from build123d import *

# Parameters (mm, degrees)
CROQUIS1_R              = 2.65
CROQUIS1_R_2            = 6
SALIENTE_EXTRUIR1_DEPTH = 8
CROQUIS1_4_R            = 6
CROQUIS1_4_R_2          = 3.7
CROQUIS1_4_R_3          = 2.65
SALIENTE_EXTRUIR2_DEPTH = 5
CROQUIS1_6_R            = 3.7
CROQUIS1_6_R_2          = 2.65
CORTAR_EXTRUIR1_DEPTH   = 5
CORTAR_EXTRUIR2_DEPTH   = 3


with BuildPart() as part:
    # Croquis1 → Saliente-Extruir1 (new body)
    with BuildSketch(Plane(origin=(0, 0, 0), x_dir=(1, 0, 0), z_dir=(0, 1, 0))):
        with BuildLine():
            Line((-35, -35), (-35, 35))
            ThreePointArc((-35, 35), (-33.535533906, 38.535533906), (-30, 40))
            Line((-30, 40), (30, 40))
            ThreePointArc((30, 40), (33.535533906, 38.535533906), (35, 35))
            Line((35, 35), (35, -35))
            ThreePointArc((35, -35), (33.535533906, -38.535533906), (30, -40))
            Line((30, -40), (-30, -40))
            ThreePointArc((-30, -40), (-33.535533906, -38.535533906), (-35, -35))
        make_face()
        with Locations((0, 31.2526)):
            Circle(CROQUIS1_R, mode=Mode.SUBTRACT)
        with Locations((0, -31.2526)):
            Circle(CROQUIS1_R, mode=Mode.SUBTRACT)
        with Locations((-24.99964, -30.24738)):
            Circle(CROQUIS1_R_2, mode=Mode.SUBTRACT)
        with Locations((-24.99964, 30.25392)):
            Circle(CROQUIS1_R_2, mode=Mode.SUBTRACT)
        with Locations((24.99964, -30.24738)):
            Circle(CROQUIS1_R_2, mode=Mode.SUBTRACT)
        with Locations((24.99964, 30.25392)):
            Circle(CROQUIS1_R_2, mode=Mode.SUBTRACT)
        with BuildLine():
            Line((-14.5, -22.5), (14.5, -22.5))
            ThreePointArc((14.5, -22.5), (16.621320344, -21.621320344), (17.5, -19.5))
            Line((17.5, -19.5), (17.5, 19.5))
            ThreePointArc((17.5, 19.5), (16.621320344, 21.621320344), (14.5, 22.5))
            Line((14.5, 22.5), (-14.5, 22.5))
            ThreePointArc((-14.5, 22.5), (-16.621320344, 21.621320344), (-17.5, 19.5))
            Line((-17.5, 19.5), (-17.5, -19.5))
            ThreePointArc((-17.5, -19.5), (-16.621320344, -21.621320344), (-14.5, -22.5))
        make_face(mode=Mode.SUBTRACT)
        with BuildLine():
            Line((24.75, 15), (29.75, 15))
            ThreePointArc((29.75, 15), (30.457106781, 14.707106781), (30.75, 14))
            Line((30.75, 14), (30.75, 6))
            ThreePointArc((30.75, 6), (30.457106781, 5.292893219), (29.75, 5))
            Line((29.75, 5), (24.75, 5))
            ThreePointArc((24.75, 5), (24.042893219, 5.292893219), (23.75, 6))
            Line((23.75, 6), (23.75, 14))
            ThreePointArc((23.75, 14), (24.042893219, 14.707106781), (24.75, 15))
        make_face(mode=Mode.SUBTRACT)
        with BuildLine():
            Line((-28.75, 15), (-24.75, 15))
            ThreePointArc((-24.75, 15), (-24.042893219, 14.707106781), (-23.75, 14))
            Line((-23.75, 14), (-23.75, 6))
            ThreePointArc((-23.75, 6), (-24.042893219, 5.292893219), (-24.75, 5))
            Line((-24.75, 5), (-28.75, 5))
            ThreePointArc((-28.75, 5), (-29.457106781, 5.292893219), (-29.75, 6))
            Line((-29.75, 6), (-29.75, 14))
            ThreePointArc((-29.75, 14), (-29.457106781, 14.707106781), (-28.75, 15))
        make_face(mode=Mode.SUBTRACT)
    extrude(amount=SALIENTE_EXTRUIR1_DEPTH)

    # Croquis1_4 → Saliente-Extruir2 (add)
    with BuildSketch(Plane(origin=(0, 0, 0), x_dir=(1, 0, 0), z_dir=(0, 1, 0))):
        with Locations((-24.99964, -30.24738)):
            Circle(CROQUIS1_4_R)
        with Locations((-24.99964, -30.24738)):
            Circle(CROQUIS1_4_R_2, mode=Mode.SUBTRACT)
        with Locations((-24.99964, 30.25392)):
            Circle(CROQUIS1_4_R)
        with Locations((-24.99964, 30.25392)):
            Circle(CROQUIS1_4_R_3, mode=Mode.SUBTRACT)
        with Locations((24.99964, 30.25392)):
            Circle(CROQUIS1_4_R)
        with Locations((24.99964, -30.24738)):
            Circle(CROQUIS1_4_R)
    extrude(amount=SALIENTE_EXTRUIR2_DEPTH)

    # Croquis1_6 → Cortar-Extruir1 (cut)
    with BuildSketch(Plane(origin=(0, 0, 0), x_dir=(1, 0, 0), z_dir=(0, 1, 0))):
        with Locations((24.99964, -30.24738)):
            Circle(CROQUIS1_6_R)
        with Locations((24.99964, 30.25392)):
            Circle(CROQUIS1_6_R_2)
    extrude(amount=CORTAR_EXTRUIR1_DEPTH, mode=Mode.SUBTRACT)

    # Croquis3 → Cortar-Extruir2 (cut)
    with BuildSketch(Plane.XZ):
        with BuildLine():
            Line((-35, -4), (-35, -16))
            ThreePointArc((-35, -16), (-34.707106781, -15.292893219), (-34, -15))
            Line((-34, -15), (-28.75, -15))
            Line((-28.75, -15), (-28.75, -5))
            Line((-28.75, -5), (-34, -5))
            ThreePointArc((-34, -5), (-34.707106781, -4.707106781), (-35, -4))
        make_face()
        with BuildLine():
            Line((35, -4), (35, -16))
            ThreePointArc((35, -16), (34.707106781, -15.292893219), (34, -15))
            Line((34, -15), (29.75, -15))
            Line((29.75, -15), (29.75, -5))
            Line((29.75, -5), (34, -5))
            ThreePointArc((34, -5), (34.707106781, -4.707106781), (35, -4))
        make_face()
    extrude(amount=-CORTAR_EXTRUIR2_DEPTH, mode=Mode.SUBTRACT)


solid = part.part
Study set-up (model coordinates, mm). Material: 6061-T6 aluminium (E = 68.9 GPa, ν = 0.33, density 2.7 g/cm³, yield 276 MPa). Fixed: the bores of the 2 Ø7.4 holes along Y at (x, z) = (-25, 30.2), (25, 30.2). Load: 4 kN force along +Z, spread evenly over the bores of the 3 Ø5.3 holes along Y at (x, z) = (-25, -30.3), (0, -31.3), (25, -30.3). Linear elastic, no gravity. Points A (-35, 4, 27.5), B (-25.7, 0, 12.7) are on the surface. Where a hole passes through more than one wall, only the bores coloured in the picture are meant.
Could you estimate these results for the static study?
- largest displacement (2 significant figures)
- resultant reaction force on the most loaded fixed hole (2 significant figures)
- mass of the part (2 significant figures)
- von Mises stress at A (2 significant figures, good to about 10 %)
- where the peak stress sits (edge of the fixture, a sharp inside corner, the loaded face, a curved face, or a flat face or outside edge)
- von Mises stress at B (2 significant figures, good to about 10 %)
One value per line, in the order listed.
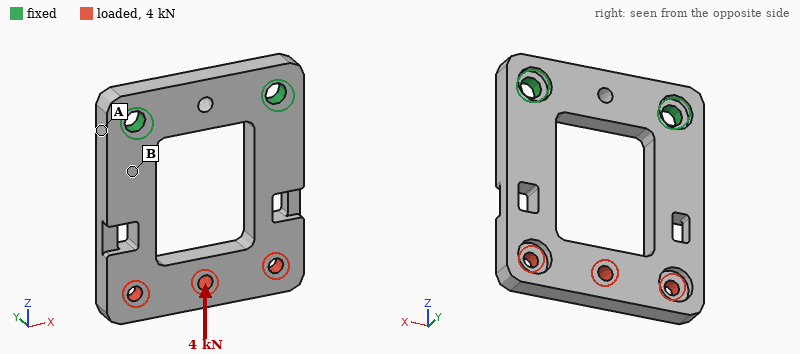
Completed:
94 µm
2.0 kN
77 g
10 MPa
a curved face
24 MPa
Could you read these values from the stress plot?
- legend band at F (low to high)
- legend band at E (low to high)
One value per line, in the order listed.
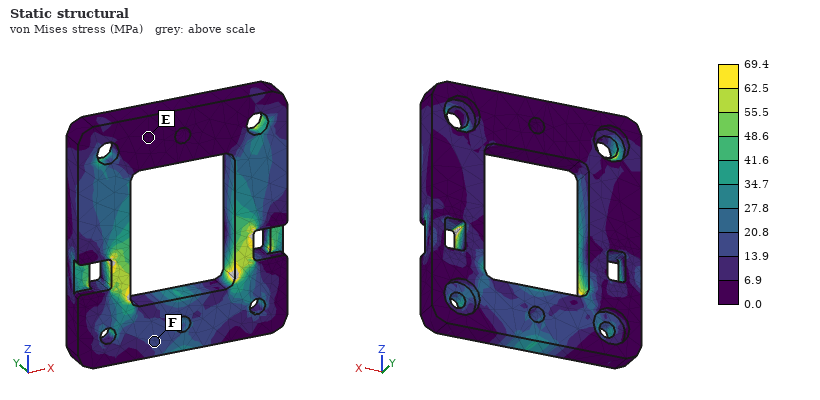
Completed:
13.9 to 20.8 MPa
0.0 to 6.9 MPa
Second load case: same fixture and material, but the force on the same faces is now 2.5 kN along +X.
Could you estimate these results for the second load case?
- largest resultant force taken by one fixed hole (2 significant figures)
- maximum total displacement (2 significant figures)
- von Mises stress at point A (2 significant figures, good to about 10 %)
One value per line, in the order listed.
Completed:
2.5 kN
0.21 mm
61 MPa
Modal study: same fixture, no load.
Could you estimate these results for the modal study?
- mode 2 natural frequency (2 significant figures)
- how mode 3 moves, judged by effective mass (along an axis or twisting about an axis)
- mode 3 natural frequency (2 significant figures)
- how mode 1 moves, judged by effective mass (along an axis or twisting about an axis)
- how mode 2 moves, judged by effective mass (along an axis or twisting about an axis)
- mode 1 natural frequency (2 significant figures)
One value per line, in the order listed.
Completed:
2200 Hz
along X
3300 Hz
along Y
twisting about Z
970 Hz
